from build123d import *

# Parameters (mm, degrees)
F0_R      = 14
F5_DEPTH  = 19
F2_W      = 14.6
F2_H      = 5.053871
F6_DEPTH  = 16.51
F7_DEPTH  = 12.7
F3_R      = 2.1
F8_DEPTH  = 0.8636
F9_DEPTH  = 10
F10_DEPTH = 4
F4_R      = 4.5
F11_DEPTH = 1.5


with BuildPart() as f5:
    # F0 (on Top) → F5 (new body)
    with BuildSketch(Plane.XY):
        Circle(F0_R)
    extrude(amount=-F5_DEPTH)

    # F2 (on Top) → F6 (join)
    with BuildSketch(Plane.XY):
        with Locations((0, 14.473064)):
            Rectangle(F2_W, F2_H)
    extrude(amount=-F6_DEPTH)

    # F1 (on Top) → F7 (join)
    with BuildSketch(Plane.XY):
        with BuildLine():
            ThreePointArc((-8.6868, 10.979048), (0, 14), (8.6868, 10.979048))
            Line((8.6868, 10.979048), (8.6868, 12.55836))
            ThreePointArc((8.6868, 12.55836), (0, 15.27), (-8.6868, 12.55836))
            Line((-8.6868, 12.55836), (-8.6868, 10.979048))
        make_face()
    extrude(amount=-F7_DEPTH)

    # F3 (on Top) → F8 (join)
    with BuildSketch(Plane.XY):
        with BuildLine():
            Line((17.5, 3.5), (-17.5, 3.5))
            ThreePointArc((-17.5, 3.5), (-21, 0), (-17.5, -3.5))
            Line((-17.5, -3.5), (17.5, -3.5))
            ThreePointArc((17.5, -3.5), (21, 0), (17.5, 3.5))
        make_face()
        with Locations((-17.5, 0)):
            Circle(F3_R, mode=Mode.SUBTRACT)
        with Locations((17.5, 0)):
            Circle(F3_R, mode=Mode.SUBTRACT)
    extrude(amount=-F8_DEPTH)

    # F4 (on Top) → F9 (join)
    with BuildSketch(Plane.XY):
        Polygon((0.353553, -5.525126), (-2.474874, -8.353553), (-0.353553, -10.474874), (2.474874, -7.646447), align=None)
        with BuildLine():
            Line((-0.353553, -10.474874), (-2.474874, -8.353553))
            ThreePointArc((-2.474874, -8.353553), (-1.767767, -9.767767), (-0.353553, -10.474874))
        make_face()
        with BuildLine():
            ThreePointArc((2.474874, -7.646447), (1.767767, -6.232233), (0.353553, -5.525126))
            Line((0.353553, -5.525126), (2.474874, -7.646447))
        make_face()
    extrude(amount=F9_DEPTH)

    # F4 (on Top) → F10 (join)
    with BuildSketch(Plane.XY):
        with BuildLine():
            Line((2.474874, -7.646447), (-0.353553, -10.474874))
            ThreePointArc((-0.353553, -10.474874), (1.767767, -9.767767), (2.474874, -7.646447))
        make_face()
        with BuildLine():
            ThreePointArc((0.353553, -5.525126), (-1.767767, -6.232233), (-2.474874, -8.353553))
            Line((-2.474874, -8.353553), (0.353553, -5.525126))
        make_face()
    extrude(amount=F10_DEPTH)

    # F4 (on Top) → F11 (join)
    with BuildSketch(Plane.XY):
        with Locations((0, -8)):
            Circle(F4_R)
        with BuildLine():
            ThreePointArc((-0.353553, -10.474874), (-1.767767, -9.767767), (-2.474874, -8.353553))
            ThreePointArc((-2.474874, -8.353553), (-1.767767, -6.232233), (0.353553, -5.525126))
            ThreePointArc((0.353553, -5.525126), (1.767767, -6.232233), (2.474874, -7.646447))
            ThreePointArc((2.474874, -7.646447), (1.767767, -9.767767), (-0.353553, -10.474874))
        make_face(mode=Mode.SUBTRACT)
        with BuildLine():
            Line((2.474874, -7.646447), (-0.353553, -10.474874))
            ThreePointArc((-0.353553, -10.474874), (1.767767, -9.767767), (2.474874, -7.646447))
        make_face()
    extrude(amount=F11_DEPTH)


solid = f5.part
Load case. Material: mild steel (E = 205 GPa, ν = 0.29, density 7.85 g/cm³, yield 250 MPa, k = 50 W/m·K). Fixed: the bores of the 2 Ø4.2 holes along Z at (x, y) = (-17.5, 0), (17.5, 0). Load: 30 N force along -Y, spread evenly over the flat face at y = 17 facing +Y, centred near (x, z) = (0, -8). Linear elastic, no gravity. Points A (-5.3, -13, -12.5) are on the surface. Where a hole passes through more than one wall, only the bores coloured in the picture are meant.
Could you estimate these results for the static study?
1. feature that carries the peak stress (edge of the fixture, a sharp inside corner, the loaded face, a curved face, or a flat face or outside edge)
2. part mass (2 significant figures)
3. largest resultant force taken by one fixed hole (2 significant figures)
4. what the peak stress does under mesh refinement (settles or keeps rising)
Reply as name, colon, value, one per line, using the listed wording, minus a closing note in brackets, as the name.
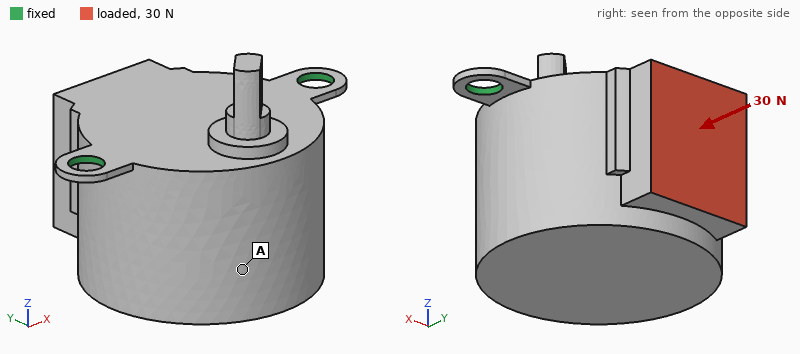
feature that carries the peak stress: edge of the fixture
part mass: 100 g
largest resultant force taken by one fixed hole: 15 N
what the peak stress does under mesh refinement: keeps rising
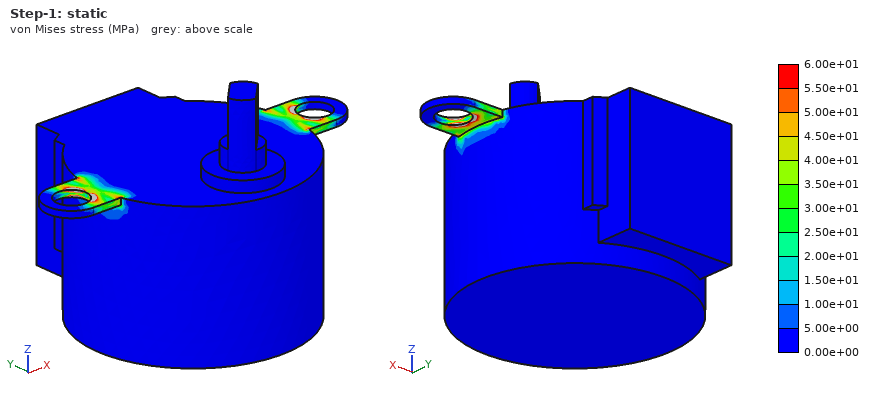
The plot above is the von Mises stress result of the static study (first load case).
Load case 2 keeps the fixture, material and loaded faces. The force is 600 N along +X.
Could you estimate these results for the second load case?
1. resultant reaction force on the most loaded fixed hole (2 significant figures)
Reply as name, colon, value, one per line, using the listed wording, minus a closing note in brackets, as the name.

resultant reaction force on the most loaded fixed hole: 470 N
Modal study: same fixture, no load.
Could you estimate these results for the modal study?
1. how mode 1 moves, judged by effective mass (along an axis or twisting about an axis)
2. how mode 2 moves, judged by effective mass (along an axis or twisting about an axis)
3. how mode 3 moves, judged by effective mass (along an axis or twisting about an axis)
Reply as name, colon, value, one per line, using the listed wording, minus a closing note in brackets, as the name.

how mode 1 moves, judged by effective mass: along Y
how mode 2 moves, judged by effective mass: along Z
how mode 3 moves, judged by effective mass: along X
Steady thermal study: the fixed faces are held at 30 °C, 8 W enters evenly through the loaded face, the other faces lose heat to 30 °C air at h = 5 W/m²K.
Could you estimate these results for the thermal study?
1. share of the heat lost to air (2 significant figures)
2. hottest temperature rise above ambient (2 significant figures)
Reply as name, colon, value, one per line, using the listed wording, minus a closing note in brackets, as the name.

share of the heat lost to air: 8.3 %
hottest temperature rise above ambient: 50 K
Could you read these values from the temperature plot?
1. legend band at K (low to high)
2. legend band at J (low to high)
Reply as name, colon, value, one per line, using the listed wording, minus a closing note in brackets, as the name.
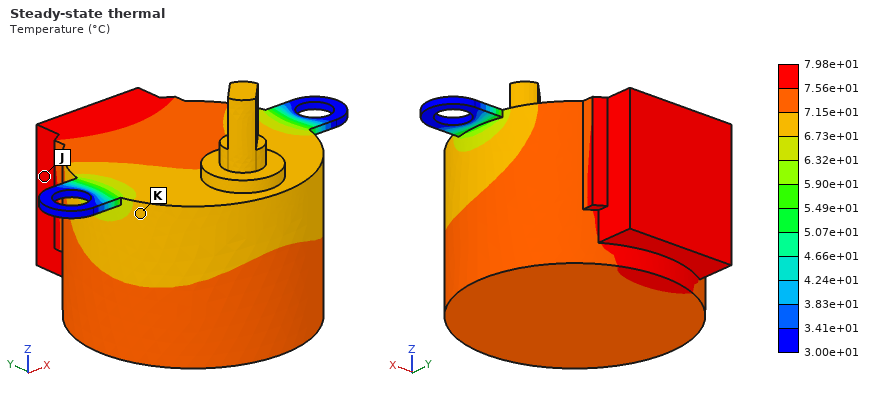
legend band at K: 6.73e+01 to 7.15e+01 °C
legend band at J: 7.56e+01 to 7.98e+01 °C
